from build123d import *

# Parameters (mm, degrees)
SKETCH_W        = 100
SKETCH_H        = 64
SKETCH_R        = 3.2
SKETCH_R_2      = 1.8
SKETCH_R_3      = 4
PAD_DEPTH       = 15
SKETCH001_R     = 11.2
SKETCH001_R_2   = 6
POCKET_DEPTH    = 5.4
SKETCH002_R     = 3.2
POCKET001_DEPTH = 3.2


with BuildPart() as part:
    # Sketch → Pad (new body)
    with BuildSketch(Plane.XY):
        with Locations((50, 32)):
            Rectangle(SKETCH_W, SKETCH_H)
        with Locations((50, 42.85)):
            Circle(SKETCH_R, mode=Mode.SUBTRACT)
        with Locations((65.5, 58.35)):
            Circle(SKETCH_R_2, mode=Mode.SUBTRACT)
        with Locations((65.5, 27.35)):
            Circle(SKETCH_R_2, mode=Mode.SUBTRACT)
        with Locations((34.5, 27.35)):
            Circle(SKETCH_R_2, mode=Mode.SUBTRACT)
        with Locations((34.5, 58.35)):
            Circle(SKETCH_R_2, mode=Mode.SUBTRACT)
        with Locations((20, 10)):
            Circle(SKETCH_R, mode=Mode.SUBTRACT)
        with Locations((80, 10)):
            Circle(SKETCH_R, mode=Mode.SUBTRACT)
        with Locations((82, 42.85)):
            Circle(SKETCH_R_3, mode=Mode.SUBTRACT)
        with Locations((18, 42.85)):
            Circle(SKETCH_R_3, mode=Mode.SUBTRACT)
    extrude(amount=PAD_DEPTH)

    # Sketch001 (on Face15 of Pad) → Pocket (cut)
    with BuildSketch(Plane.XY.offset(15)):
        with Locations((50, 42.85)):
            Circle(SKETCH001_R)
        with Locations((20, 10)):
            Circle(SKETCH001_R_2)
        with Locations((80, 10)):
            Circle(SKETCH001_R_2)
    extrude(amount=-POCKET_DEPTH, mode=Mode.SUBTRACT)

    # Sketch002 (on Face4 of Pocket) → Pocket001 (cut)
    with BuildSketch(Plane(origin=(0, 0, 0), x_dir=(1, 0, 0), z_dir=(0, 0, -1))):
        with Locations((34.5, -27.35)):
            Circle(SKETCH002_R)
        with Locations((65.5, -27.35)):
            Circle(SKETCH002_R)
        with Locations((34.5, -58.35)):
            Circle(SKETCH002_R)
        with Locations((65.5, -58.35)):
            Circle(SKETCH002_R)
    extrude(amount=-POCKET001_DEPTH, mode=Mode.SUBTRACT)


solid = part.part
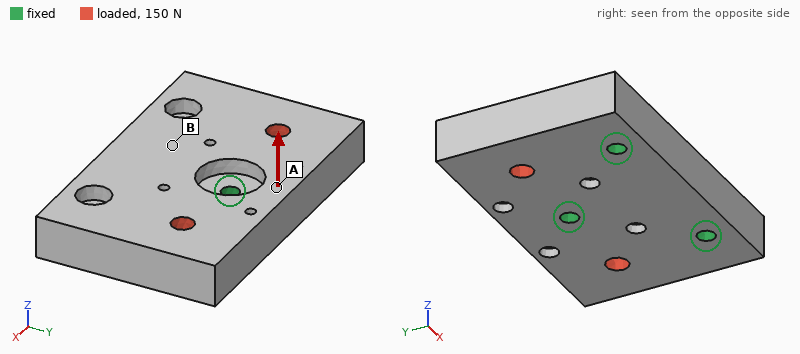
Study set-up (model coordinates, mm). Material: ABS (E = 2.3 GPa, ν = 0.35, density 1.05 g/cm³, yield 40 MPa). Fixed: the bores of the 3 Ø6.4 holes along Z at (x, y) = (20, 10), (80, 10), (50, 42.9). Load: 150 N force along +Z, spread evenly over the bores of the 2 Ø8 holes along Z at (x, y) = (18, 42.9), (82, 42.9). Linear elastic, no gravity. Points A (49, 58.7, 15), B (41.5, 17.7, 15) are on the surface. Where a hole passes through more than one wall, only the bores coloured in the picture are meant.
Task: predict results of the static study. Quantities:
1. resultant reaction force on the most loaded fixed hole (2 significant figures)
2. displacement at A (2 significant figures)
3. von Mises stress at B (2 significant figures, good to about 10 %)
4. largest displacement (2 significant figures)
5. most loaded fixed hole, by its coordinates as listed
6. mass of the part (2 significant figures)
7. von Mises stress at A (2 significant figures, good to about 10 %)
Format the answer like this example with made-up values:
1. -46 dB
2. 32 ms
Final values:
1. 100 N
2. 10 µm
3. 0.34 MPa
4. 49 µm
5. (50, 42.9)
6. 94 g
7. 1.0 MPa
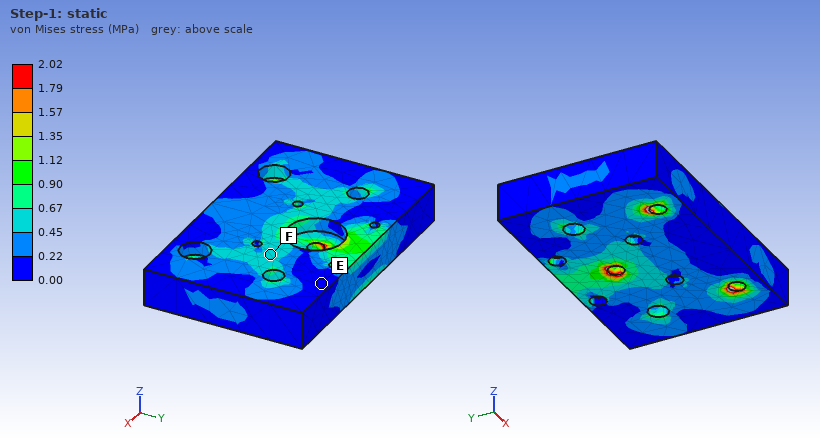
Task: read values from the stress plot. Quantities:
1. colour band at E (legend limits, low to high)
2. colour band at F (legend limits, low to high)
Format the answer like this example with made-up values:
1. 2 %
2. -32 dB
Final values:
1. 0.00 to 0.22 MPa
2. 0.45 to 0.67 MPa
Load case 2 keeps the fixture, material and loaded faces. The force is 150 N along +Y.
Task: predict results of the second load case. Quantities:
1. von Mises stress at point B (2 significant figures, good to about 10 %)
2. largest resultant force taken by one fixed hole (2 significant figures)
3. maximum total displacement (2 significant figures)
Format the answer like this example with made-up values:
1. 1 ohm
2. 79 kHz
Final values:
1. 0.058 MPa
2. 54 N
3. 4.3 µm
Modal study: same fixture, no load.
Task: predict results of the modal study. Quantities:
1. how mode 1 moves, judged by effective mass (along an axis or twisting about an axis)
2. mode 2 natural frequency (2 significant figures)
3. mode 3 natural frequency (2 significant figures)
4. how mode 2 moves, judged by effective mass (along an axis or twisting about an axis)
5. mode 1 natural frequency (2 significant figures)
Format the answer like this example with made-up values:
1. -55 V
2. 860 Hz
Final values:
1. twisting about Y
2. 1600 Hz
3. 3800 Hz
4. along Z
5. 1500 Hz
